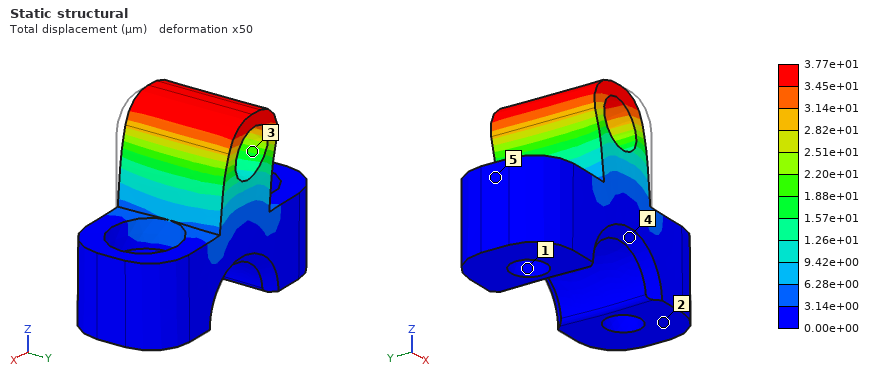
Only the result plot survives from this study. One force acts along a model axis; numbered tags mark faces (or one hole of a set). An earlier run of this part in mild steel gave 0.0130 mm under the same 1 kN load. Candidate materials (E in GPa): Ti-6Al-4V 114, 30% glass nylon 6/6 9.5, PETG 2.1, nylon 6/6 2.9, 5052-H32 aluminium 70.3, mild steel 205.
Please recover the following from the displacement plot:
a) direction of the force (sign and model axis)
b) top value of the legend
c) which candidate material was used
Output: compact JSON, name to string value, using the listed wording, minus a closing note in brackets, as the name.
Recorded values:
{"direction of the force": "-X", "top value of the legend": "3.77e+01 µm", "which candidate material was used": "5052-H32 aluminium"}
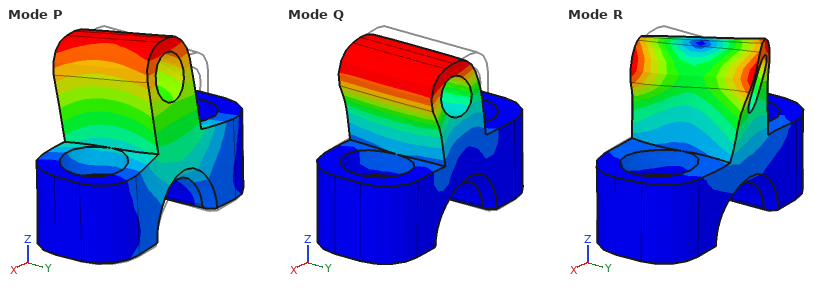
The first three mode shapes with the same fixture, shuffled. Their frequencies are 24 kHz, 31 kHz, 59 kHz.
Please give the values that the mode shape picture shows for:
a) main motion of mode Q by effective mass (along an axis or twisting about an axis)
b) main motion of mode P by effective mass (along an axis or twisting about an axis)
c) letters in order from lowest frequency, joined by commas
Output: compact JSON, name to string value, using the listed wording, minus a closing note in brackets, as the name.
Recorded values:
{"main motion of mode Q by effective mass": "along X", "main motion of mode P by effective mass": "along Y", "letters in order from lowest frequency, joined by commas": "P, Q, R"}
